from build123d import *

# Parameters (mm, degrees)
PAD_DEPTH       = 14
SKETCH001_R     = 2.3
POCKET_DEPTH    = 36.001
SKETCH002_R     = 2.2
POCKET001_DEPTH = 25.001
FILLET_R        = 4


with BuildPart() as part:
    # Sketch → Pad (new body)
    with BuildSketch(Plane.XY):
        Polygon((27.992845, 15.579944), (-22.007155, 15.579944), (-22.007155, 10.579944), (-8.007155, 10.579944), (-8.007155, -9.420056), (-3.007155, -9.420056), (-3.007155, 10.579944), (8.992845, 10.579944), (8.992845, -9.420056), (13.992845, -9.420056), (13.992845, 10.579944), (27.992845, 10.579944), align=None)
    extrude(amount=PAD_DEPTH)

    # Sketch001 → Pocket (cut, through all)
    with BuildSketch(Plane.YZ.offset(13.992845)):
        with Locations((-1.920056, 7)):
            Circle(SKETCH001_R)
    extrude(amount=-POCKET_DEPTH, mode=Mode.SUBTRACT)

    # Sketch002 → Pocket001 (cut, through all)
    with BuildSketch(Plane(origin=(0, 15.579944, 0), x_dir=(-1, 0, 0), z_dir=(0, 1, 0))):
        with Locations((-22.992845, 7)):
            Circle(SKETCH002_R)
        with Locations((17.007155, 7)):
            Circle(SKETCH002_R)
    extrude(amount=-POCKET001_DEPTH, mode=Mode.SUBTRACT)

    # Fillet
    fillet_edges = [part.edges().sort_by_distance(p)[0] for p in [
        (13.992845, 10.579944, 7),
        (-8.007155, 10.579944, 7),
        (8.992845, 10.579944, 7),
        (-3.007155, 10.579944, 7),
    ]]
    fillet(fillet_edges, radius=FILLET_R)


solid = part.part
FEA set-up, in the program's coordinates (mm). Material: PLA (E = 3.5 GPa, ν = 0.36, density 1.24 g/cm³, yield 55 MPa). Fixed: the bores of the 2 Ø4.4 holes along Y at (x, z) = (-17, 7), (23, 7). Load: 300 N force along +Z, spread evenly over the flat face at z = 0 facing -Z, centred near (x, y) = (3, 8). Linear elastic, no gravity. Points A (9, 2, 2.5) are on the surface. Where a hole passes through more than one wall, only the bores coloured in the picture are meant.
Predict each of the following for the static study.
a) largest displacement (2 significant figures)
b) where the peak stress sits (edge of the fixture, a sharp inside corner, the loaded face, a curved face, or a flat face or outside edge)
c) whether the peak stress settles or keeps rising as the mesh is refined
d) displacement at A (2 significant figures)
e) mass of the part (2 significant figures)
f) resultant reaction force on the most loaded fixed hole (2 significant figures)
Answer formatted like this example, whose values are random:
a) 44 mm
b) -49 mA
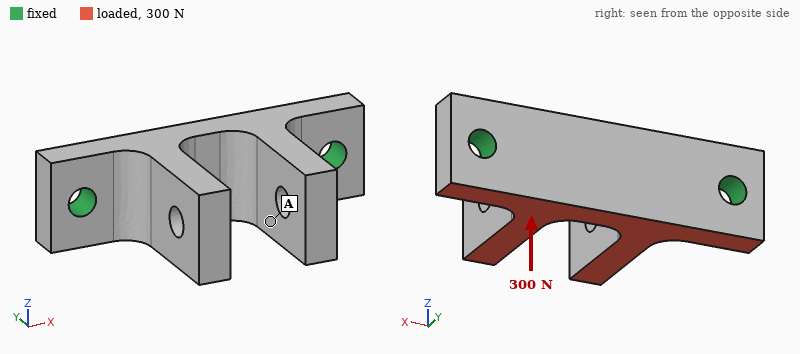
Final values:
a) 0.27 mm
b) edge of the fixture
c) keeps rising
d) 0.14 mm
e) 7.7 g
f) 150 N
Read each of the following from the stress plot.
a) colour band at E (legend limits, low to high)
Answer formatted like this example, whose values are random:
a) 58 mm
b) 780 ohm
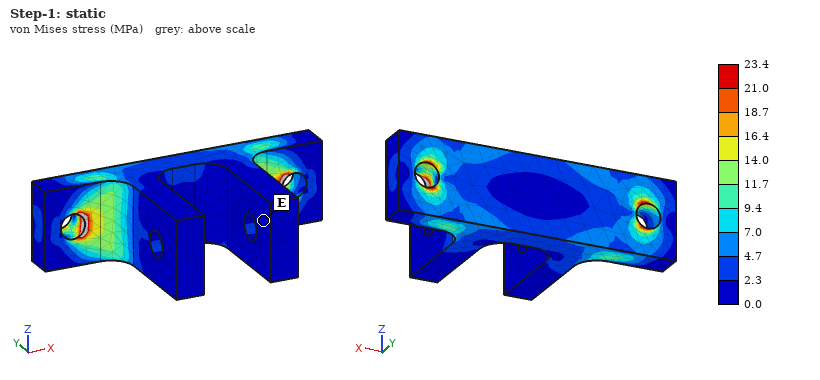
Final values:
a) 0.0 to 2.3 MPa
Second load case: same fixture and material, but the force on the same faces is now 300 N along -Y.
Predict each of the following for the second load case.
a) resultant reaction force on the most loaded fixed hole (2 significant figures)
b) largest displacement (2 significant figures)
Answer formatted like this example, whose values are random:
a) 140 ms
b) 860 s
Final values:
a) 150 N
b) 0.30 mm
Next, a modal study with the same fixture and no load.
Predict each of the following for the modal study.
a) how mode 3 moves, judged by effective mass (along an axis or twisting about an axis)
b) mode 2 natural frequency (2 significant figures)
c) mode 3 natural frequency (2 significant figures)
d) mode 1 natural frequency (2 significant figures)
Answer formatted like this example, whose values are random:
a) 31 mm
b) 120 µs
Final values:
a) along X
b) 2400 Hz
c) 3400 Hz
d) 2300 Hz
